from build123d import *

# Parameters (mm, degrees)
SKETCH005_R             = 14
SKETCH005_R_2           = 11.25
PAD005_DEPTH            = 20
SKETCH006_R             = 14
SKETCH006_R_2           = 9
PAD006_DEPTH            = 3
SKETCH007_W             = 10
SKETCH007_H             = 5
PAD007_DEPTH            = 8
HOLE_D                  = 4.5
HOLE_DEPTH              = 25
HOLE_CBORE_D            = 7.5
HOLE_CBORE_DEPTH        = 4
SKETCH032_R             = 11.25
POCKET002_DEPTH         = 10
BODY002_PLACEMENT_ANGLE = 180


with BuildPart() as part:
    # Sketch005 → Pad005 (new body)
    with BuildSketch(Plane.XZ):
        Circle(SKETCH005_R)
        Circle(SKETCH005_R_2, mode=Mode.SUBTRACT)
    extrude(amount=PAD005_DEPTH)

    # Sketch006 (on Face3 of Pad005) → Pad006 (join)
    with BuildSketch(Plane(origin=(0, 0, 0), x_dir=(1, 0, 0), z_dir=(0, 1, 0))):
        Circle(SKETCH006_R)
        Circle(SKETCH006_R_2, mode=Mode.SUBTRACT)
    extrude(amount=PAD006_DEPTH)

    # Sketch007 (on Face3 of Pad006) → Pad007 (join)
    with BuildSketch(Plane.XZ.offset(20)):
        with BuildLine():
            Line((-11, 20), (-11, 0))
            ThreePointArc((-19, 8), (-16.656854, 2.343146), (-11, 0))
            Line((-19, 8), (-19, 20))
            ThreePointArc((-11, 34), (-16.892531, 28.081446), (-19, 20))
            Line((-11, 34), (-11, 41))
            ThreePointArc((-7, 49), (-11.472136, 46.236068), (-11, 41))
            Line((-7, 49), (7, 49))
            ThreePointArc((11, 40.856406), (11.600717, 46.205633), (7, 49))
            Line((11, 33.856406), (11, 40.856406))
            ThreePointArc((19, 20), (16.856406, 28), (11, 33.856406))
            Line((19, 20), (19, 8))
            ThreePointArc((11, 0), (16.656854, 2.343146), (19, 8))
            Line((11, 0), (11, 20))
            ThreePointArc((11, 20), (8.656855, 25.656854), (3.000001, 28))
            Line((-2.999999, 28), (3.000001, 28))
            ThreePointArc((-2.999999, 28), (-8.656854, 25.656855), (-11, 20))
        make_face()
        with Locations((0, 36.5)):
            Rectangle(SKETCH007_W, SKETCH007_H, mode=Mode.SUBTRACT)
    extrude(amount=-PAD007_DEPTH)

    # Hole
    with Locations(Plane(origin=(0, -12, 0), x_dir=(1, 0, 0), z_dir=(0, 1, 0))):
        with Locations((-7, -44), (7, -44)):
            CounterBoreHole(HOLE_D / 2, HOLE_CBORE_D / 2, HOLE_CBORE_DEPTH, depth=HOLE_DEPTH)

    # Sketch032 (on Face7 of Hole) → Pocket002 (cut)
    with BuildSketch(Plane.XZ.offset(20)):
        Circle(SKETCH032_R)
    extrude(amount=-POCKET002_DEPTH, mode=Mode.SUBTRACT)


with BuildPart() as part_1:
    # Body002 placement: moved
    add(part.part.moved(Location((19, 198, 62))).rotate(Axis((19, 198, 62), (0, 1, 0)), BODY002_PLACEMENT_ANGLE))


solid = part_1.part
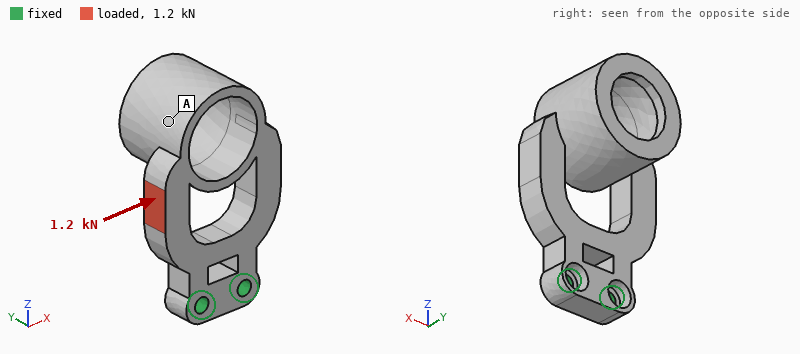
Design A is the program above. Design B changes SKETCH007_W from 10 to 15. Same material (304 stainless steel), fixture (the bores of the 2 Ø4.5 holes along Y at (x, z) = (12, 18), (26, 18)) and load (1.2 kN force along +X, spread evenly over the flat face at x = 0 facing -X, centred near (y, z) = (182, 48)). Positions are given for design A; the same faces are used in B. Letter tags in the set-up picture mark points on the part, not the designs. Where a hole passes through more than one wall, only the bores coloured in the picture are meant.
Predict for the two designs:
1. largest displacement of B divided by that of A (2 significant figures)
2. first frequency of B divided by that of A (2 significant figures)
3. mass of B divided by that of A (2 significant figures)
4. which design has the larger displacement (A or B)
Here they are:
1.2
0.85
0.98
B
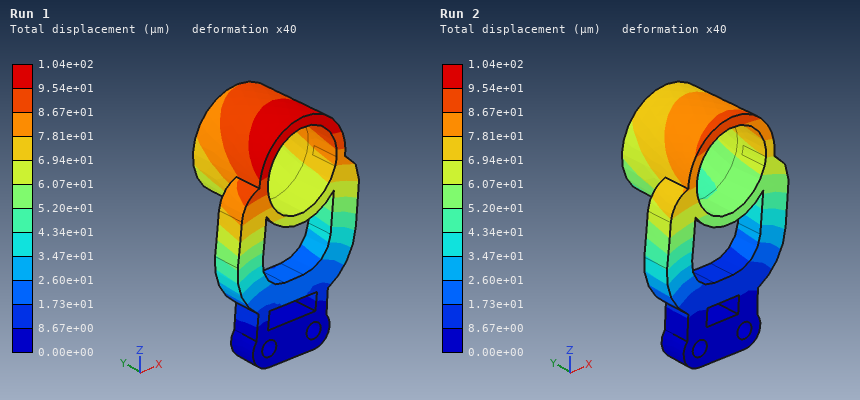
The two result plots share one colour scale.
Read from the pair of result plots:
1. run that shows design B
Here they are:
Run 1
